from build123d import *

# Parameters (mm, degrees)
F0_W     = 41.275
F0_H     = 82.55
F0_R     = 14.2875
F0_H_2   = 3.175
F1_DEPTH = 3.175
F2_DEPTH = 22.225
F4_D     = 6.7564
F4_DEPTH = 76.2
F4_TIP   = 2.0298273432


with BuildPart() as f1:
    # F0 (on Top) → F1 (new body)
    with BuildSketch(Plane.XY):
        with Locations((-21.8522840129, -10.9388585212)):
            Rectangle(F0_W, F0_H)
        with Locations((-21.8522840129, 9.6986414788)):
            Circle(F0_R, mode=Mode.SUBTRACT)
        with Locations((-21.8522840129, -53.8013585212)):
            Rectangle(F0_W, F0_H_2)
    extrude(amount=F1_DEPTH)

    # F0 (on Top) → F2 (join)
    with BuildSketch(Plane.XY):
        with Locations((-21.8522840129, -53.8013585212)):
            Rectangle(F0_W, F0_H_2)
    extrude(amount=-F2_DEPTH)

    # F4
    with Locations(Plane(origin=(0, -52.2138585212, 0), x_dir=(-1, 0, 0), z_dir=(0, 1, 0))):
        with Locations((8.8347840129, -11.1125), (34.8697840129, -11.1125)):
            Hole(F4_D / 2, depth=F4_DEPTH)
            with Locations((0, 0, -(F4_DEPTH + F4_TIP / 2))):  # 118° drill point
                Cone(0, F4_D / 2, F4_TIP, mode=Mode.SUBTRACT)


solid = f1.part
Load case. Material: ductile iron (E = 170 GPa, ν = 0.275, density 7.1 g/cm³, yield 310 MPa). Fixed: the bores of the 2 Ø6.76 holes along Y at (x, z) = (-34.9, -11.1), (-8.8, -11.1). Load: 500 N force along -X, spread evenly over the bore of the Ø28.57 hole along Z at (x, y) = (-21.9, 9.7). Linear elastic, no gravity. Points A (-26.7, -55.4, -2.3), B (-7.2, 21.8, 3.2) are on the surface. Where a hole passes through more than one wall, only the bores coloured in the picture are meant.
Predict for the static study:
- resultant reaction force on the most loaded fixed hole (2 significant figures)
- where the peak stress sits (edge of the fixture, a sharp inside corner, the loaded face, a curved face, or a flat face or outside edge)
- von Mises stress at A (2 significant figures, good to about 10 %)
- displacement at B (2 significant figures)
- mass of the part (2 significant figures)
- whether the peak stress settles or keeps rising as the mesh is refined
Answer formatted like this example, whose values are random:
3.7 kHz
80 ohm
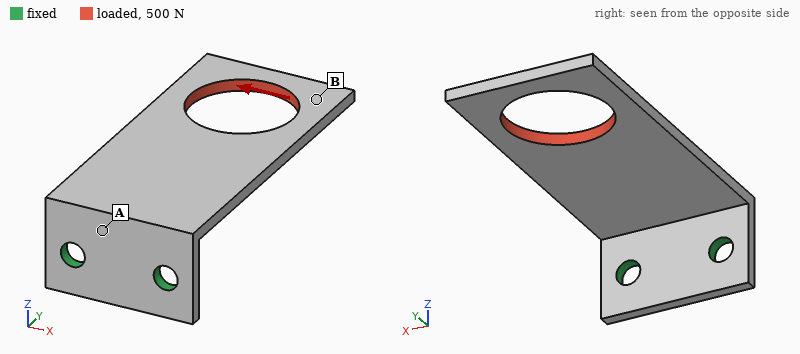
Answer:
1.1 kN
edge of the fixture
92 MPa
0.21 mm
84 g
keeps rising
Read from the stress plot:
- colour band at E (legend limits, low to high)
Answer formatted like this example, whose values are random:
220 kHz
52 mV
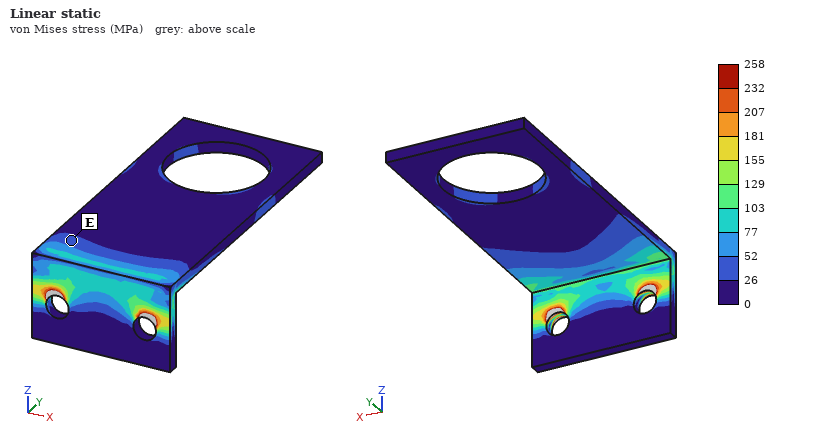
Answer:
26 to 52 MPa
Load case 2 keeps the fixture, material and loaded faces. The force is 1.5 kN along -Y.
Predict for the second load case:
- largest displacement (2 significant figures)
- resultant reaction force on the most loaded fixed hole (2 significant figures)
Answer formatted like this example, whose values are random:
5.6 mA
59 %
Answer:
0.40 mm
750 N
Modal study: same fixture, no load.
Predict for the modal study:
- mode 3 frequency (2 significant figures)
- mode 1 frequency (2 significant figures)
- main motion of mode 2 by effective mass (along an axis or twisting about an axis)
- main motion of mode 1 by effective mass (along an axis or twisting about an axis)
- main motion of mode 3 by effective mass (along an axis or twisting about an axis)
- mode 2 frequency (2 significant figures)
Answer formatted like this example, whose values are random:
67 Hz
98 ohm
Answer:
1600 Hz
360 Hz
along X
along Z
along X
1300 Hz
